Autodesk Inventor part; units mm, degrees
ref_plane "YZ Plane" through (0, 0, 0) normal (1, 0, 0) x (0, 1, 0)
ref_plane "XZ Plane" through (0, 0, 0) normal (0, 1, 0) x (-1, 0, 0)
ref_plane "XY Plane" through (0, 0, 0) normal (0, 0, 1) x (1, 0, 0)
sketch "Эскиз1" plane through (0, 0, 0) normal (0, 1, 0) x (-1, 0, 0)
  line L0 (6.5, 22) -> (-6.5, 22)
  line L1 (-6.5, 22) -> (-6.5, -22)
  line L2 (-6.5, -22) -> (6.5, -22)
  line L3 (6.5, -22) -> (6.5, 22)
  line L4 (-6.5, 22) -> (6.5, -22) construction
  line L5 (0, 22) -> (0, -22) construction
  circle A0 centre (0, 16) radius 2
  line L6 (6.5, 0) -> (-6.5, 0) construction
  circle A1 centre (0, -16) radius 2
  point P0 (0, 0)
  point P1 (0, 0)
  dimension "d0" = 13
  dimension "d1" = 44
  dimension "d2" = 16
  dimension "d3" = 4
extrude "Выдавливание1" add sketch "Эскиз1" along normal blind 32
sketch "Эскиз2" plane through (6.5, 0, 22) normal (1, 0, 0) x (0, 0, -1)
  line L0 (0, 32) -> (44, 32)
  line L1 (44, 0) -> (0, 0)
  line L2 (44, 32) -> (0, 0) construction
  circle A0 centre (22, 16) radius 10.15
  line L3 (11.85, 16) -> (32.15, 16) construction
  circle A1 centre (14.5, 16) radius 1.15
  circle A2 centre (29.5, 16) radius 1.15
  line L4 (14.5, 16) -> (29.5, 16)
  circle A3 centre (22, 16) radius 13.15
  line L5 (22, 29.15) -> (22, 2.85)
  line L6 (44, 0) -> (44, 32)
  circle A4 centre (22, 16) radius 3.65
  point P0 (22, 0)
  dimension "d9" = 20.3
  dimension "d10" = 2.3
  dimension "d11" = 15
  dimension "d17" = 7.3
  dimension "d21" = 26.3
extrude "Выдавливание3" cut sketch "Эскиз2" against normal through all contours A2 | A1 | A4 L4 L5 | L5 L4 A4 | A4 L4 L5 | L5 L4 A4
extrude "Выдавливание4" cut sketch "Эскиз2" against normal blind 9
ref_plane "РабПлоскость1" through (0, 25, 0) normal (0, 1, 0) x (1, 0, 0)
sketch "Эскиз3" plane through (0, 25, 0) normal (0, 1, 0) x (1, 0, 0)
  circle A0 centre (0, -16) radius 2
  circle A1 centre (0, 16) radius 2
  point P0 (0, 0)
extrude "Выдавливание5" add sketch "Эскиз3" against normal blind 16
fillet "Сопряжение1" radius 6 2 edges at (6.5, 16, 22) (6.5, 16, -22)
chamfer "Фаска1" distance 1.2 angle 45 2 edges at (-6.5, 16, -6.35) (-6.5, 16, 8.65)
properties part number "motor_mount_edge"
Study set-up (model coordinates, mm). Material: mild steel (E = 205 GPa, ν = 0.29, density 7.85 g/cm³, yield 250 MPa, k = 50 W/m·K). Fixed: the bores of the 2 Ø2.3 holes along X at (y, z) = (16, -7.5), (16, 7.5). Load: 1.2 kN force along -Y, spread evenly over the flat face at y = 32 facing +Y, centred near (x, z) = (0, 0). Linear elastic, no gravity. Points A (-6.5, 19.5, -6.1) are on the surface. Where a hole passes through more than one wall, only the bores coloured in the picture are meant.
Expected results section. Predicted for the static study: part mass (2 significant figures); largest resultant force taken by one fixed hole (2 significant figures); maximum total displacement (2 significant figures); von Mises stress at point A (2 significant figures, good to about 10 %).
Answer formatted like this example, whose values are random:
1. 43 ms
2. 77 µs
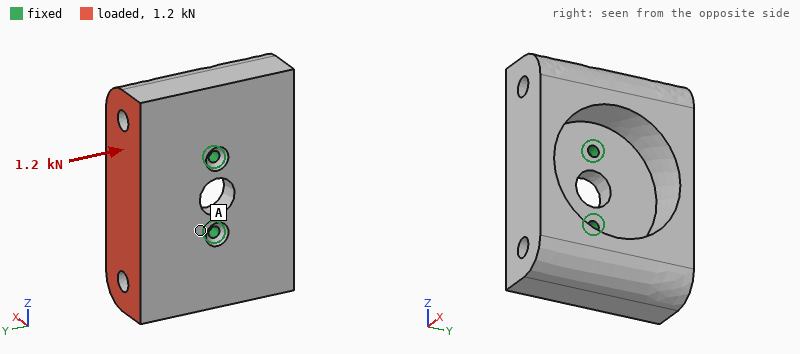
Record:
1. 97 g
2. 610 N
3. 17 µm
4. 19 MPa
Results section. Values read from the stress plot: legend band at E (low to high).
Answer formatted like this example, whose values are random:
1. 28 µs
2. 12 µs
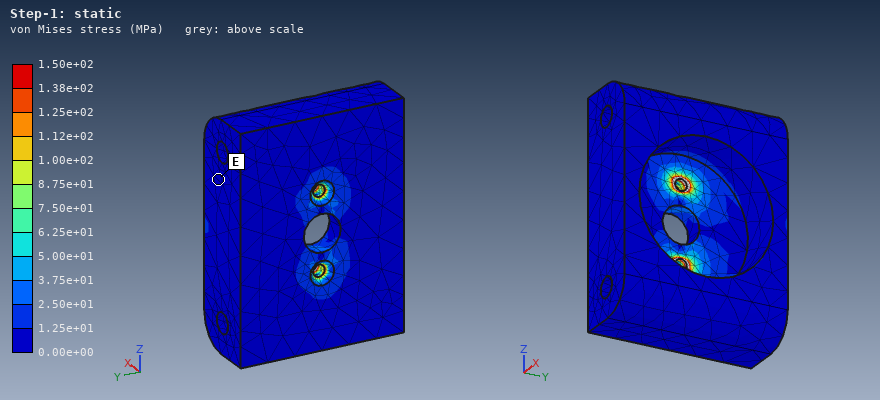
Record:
1. 0.00e+00 to 1.25e+01 MPa
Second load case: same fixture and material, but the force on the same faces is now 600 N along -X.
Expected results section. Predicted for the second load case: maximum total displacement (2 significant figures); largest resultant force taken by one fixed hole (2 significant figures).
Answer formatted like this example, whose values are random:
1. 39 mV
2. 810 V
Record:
1. 32 µm
2. 300 N
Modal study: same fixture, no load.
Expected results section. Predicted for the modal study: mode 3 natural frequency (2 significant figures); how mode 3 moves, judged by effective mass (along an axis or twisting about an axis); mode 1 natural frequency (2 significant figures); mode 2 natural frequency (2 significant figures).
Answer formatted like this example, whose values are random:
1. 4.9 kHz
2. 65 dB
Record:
1. 9900 Hz
2. twisting about X
3. 3600 Hz
4. 6600 Hz
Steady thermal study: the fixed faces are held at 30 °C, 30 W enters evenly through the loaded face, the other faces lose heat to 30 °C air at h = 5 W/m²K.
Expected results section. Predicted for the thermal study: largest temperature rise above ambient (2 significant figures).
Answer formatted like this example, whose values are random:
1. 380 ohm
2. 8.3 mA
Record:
1. 61 K
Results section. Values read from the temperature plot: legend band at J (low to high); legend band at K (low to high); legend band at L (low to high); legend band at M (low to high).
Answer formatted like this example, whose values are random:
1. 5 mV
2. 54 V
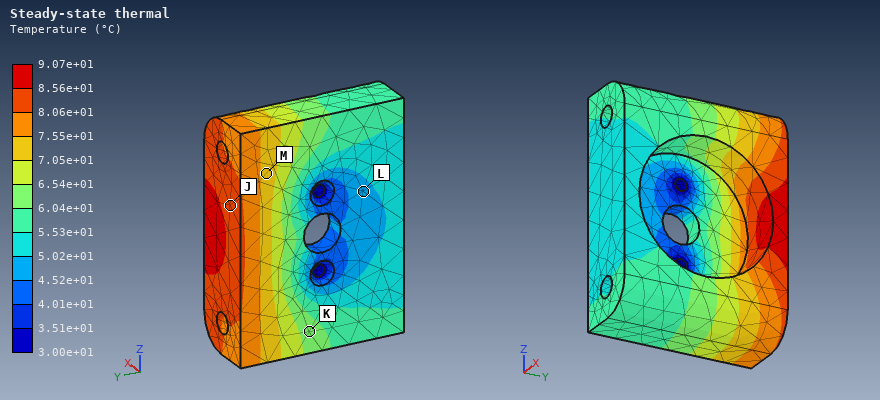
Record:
1. 8.06e+01 to 8.56e+01 °C
2. 6.04e+01 to 6.54e+01 °C
3. 4.52e+01 to 5.02e+01 °C
4. 7.05e+01 to 7.55e+01 °C
